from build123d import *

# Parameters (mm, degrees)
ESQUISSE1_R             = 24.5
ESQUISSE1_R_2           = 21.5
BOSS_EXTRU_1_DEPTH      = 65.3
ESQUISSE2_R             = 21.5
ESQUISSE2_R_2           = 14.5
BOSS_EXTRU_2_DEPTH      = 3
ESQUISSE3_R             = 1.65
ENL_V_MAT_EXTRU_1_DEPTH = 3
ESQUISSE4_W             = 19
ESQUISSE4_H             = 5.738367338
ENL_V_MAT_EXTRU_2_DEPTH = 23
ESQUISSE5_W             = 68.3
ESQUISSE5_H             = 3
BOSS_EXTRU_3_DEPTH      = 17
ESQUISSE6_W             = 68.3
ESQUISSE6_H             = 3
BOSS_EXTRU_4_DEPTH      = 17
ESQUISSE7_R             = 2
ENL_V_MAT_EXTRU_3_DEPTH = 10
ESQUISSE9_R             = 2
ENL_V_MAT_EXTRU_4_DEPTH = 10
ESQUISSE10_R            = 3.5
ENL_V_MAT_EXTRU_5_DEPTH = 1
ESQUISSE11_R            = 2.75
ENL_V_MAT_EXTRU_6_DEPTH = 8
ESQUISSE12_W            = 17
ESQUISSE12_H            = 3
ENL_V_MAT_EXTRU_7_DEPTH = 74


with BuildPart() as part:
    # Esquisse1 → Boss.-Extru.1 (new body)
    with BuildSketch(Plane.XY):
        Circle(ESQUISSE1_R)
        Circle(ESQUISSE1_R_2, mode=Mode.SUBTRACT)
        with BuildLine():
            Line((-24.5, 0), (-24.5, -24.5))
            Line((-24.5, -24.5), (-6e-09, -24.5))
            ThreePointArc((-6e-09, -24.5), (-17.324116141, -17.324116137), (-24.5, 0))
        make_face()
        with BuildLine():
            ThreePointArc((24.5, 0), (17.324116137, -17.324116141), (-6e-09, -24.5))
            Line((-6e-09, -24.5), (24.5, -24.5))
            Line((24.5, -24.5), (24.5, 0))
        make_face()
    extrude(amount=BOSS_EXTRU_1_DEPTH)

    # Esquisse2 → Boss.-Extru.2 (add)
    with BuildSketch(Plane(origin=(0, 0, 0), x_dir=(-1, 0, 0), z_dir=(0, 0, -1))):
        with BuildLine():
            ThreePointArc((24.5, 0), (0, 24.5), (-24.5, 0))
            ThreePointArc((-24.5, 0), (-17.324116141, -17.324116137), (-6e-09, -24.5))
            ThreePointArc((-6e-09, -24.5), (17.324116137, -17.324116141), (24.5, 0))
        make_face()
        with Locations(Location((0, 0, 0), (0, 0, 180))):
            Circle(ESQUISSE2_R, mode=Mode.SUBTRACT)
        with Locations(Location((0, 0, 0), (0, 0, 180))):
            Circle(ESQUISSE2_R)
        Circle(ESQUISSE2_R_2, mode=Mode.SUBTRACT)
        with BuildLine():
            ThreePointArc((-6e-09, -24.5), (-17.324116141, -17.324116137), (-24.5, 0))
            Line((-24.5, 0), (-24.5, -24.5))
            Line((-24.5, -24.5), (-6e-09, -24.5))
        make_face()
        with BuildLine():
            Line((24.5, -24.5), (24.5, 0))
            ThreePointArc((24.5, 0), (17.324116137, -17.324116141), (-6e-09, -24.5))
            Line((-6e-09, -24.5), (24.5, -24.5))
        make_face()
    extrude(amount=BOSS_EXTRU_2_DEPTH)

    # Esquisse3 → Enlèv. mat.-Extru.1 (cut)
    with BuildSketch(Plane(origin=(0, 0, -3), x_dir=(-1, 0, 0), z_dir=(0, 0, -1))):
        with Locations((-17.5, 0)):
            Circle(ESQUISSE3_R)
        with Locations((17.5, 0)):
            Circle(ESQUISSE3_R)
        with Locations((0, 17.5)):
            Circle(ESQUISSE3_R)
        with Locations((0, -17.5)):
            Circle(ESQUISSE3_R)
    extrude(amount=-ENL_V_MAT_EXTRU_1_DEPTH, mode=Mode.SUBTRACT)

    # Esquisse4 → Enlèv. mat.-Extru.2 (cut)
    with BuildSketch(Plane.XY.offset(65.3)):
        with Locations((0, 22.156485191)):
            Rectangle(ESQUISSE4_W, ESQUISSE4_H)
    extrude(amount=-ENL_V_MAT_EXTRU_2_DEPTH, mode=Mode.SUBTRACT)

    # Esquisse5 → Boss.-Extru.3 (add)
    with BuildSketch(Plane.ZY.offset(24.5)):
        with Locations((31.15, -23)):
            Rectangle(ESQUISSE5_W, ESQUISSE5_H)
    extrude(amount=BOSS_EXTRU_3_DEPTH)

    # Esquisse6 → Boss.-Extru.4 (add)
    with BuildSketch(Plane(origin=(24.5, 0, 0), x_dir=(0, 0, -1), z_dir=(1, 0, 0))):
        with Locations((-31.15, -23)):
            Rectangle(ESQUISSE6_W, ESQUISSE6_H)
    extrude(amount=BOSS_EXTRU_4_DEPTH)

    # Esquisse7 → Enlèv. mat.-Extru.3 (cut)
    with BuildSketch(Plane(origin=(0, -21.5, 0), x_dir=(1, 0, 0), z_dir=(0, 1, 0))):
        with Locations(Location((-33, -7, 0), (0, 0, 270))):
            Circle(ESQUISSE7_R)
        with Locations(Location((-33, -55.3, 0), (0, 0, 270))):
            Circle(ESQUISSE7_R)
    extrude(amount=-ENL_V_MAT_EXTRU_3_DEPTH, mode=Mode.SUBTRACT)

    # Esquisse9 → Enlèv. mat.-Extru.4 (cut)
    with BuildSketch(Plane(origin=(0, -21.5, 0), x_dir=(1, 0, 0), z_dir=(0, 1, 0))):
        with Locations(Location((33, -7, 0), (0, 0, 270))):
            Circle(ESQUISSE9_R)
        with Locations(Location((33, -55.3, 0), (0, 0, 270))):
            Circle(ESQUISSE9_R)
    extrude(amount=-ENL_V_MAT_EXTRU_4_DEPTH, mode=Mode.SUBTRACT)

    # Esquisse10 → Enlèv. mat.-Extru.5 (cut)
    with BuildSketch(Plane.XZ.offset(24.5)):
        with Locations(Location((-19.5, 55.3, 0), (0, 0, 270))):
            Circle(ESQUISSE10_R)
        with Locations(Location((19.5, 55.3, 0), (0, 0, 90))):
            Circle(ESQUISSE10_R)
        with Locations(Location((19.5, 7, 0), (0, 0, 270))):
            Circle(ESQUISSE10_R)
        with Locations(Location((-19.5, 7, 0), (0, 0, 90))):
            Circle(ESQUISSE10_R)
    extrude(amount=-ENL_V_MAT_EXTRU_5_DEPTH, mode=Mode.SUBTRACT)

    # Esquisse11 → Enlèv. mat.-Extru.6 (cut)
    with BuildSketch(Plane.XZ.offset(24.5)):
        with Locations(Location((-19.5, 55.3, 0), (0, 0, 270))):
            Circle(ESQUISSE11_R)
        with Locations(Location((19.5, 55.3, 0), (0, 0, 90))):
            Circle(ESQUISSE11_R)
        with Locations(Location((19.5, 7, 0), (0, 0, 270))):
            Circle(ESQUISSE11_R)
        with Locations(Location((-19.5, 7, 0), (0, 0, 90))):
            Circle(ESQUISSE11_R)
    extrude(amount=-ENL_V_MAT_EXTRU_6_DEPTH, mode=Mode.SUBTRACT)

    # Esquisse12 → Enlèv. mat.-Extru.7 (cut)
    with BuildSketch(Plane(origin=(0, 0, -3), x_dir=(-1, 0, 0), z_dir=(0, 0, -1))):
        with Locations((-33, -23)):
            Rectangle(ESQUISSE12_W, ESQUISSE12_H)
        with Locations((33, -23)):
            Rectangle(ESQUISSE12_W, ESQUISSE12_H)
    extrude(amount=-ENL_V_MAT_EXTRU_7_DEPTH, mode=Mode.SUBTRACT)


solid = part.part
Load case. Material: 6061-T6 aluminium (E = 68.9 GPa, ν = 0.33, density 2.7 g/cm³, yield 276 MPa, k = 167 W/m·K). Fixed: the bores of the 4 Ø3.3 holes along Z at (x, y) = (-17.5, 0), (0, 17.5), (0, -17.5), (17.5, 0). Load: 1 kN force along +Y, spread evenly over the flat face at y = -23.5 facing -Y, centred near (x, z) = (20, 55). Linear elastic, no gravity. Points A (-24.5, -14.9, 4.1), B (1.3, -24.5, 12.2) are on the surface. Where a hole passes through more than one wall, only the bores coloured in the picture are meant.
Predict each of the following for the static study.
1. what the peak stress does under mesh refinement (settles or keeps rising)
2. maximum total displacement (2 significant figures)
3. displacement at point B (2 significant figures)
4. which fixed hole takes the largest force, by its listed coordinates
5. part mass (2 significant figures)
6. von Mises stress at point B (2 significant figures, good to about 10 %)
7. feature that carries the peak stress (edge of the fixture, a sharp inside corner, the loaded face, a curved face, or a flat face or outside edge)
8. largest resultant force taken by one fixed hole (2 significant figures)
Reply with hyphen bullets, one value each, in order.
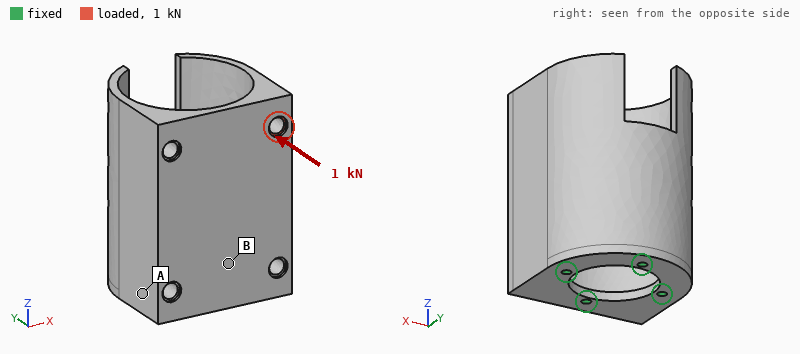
- keeps rising
- 0.13 mm
- 0.036 mm
- (0, -17.5)
- 130 g
- 22 MPa
- edge of the fixture
- 1.5 kN
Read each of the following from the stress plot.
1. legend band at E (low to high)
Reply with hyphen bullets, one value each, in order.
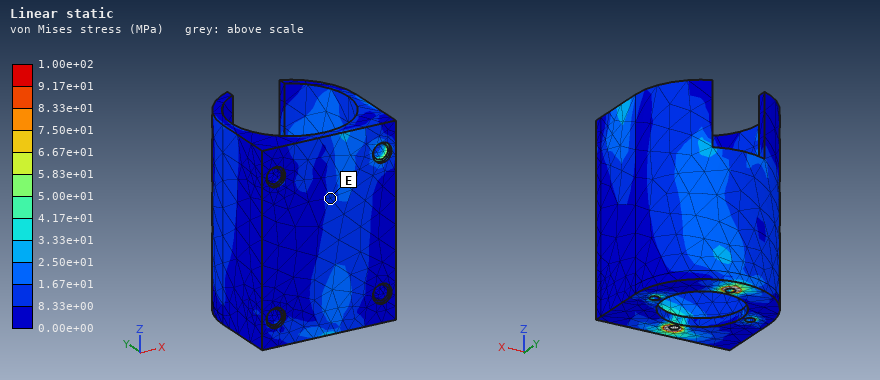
- 8.33e+00 to 1.67e+01 MPa
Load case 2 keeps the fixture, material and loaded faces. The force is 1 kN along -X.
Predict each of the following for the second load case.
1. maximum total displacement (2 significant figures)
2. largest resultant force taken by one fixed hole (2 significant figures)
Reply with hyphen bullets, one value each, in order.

- 0.11 mm
- 1.4 kN
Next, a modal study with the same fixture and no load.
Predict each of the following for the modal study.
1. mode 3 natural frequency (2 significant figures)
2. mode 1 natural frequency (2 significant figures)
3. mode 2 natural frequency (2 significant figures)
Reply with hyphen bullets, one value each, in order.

- 4100 Hz
- 2300 Hz
- 2300 Hz
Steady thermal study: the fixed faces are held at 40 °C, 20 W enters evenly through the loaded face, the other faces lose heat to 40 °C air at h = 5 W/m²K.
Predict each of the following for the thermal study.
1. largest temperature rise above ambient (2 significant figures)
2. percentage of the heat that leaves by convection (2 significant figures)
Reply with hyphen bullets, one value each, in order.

- 31 K
- 5.0 %
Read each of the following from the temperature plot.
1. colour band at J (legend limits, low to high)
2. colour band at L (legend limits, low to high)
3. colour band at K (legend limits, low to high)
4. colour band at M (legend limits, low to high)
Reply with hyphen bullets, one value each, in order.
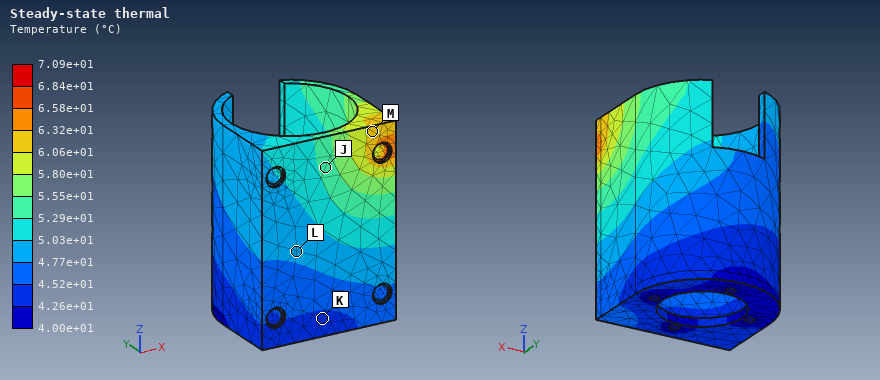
- 5.29e+01 to 5.55e+01 °C
- 4.77e+01 to 5.03e+01 °C
- 4.26e+01 to 4.52e+01 °C
- 6.06e+01 to 6.32e+01 °C
